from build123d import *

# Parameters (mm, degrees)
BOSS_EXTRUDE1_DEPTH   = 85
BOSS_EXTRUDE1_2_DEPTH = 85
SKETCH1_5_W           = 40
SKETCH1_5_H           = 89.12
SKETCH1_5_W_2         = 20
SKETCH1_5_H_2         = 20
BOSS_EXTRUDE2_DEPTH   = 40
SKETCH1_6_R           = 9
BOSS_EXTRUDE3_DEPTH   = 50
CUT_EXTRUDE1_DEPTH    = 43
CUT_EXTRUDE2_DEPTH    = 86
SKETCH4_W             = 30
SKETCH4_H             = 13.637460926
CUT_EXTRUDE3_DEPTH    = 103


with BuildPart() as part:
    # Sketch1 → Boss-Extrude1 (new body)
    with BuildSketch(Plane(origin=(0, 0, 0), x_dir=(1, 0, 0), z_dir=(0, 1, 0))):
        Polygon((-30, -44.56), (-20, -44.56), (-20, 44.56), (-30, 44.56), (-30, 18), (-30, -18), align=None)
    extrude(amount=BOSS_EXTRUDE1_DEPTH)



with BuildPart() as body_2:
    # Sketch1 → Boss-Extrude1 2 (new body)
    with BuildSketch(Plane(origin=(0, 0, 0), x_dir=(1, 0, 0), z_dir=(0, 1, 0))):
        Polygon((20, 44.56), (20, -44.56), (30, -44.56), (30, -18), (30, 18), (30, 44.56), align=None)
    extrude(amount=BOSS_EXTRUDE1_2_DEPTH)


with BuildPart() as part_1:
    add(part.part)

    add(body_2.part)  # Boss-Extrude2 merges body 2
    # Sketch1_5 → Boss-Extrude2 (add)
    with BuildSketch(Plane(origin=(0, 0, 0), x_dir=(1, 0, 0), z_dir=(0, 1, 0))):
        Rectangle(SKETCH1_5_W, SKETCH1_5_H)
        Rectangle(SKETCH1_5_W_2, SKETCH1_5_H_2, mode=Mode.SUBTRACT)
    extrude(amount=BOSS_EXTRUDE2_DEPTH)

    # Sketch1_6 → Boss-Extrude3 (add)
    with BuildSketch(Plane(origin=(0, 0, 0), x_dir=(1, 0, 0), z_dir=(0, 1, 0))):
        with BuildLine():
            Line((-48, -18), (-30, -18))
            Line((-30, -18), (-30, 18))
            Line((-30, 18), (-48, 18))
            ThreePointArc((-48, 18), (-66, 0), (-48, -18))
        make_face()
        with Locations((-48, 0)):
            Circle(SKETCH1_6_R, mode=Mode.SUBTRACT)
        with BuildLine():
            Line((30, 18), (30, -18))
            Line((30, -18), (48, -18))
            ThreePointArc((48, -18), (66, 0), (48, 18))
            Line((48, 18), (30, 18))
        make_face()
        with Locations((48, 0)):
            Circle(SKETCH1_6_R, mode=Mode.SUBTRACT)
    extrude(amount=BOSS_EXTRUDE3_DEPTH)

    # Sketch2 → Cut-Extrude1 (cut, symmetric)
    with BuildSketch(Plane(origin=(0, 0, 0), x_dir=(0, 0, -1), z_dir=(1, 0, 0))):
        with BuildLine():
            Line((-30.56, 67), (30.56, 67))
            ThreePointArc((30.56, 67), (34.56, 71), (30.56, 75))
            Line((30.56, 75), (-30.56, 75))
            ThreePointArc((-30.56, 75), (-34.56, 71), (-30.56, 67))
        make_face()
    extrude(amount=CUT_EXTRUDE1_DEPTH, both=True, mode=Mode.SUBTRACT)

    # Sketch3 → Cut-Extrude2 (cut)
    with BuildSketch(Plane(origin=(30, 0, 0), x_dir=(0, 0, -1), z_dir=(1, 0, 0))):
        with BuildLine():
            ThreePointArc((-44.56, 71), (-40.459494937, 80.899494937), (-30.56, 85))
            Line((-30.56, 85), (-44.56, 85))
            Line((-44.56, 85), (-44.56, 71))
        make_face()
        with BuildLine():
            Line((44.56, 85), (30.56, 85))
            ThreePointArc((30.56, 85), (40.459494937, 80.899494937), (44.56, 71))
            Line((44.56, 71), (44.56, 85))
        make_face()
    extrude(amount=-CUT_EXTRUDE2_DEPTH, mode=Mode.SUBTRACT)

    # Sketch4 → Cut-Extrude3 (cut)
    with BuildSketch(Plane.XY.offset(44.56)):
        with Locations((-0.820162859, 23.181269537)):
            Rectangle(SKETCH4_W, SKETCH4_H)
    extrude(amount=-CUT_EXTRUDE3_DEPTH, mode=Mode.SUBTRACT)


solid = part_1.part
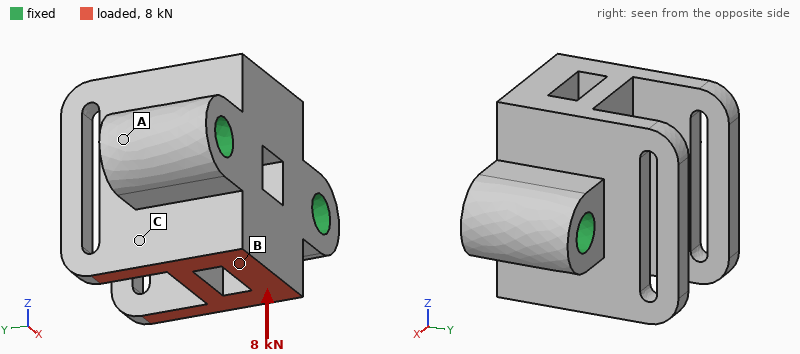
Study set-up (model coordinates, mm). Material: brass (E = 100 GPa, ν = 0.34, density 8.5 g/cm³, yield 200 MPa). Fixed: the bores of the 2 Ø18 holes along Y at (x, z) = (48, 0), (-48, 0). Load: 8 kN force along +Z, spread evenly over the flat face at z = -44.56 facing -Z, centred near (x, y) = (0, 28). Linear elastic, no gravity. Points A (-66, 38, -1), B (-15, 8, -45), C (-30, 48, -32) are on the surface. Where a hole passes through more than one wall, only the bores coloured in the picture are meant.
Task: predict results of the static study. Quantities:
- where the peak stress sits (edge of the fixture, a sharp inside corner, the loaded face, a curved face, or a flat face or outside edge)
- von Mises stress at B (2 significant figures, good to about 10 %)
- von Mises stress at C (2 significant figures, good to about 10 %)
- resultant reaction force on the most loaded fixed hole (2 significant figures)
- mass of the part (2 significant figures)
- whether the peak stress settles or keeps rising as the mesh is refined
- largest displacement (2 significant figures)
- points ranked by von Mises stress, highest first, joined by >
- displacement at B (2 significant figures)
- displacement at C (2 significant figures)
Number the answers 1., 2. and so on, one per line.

1. edge of the fixture
2. 2.9 MPa
3. 3.7 MPa
4. 4.1 kN
5. 2.8 kg
6. keeps rising
7. 3.9 µm
8. C > B > A
9. 2.4 µm
10. 2.7 µm
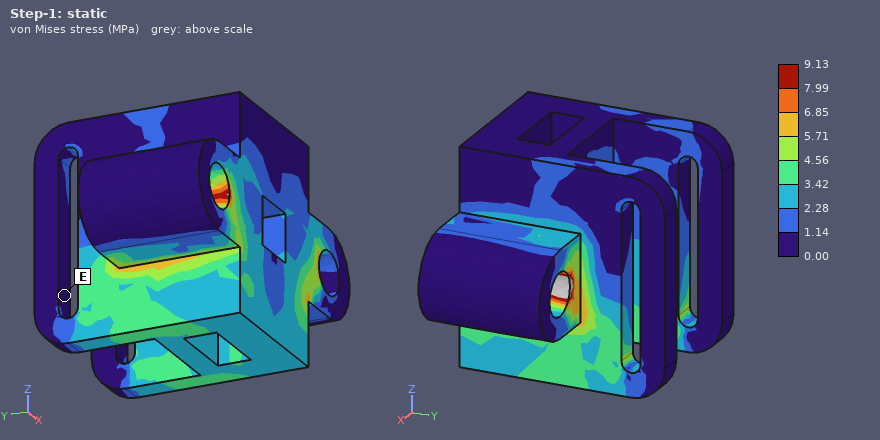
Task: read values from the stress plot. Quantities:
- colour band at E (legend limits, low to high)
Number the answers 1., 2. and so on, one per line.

1. 0.00 to 1.14 MPa
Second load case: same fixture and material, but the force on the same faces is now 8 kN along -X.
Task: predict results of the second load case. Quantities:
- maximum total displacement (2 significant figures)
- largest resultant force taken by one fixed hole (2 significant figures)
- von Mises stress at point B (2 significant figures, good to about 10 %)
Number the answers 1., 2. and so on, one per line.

1. 34 µm
2. 5.6 kN
3. 7.6 MPa
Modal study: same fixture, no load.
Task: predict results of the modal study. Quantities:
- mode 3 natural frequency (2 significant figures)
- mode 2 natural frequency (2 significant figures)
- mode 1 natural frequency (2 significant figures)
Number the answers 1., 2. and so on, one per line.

1. 3500 Hz
2. 2200 Hz
3. 2200 Hz
